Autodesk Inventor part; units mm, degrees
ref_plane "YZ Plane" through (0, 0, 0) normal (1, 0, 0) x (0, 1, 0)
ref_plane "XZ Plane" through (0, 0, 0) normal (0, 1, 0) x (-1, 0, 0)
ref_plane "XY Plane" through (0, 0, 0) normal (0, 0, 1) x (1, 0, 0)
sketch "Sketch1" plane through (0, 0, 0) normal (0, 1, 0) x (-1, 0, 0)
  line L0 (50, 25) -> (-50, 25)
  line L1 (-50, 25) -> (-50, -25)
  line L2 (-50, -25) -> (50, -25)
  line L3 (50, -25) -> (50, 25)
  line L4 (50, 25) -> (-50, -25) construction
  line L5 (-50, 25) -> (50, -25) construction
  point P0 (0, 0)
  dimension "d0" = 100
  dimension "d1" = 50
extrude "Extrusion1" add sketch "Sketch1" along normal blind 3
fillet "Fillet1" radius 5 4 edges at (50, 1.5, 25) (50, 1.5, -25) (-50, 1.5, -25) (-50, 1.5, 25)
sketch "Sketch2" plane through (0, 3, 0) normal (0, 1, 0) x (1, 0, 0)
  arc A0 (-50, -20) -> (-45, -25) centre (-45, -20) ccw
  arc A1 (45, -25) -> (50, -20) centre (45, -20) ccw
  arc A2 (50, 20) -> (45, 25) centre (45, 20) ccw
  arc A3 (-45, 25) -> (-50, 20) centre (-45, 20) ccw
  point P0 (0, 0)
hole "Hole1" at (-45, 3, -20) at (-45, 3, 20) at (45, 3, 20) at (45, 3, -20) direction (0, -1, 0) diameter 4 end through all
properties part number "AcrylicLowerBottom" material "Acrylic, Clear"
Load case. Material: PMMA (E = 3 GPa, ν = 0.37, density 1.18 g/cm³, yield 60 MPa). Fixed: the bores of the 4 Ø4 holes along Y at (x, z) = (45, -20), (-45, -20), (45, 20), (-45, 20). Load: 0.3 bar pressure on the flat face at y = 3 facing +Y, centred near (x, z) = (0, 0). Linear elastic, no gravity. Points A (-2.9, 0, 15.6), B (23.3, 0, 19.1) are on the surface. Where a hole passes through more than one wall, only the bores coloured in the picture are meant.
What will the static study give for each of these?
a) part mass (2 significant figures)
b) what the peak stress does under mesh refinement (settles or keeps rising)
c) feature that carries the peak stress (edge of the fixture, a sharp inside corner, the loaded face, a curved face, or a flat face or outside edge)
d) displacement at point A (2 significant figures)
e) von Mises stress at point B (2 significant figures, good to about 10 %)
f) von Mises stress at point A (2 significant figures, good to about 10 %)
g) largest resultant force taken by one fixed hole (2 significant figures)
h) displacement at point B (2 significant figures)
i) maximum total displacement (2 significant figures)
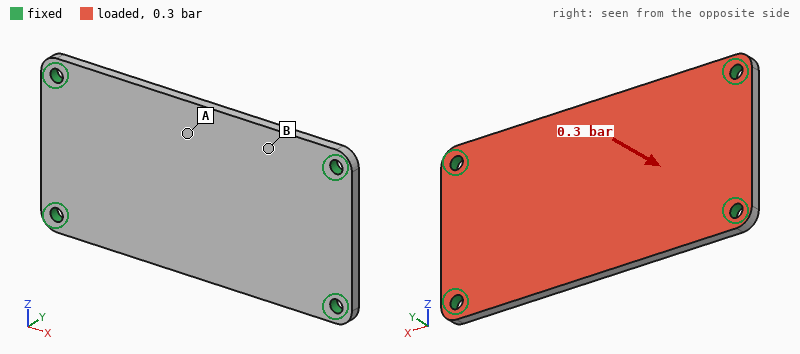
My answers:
17 g
keeps rising
edge of the fixture
0.86 mm
3.1 MPa
6.9 MPa
37 N
0.49 mm
0.91 mm
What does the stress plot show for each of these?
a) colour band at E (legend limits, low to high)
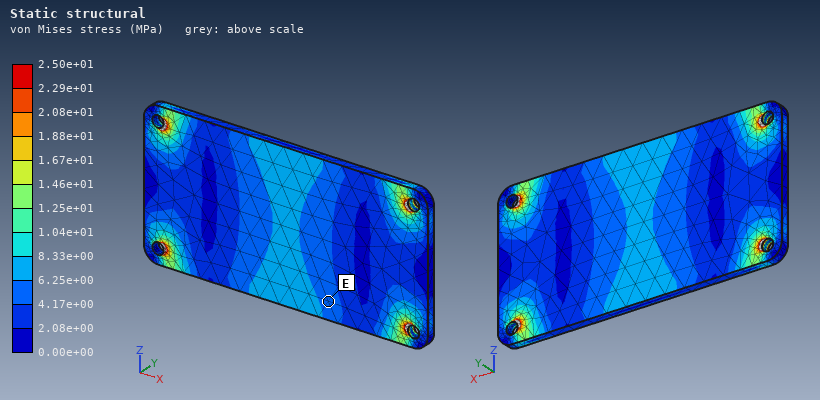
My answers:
4.17e+00 to 6.25e+00 MPa
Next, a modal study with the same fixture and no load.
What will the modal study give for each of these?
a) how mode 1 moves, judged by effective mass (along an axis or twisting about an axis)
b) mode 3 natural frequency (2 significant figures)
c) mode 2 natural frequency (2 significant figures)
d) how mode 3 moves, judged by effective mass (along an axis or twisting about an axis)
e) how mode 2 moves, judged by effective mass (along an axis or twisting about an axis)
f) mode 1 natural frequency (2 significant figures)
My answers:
along Y
1600 Hz
950 Hz
twisting about Z
twisting about X
560 Hz
